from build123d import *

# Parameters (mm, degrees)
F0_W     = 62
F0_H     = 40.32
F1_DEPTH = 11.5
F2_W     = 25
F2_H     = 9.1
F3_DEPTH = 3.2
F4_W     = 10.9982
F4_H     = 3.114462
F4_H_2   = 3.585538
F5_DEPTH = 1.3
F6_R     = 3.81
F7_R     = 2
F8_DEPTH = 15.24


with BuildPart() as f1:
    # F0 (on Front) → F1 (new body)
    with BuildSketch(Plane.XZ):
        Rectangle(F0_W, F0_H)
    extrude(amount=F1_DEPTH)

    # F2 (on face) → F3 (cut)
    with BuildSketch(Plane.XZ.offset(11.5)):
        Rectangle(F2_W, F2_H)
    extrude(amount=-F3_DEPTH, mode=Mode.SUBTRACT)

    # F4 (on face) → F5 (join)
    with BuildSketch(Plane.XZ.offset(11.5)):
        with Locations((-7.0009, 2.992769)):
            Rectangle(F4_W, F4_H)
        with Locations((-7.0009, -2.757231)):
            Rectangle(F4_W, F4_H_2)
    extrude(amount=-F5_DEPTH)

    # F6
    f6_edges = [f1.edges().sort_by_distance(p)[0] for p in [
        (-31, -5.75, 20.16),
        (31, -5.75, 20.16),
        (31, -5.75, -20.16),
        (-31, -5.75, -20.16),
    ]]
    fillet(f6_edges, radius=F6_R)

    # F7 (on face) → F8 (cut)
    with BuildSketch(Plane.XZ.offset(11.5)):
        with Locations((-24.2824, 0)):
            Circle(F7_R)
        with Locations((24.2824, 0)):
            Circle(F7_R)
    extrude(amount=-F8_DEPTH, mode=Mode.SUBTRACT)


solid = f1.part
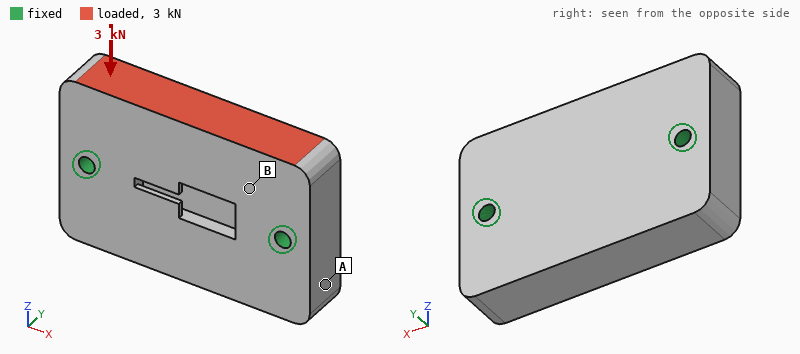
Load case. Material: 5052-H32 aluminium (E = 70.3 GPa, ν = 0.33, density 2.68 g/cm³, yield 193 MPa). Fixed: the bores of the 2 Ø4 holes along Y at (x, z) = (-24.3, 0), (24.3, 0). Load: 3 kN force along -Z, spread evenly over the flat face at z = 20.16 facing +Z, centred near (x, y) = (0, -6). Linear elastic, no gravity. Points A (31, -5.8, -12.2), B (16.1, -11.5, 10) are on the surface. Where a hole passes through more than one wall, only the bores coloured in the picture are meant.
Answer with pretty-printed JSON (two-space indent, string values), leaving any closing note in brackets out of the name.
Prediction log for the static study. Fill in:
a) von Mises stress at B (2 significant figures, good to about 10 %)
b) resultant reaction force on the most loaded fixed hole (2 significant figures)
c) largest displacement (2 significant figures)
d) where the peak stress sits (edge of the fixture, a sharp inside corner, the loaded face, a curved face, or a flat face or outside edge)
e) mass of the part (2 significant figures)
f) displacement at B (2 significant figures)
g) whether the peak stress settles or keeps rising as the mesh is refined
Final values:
{
  "von Mises stress at B": "6.8 MPa",
  "resultant reaction force on the most loaded fixed hole": "1.5 kN",
  "largest displacement": "3.8 µm",
  "where the peak stress sits": "edge of the fixture",
  "mass of the part": "74 g",
  "displacement at B": "2.0 µm",
  "whether the peak stress settles or keeps rising as the mesh is refined": "keeps rising"
}
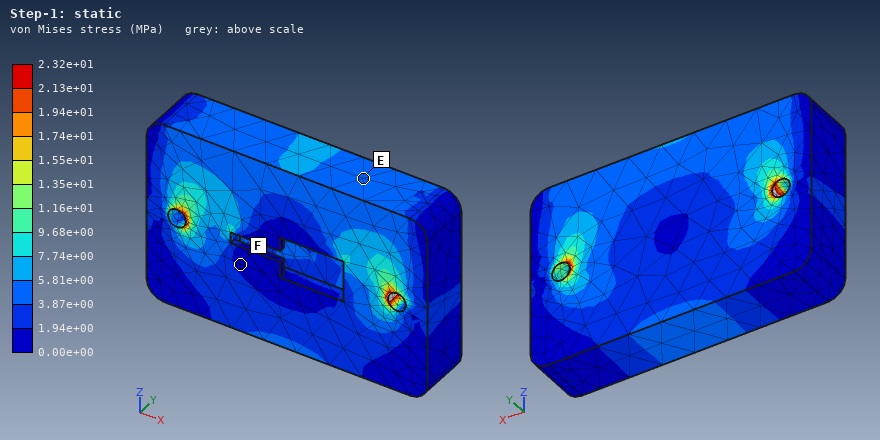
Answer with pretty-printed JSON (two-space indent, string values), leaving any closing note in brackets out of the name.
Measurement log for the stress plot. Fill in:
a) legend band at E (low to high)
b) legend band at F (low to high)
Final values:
{
  "legend band at E": "3.87e+00 to 5.81e+00 MPa",
  "legend band at F": "0.00e+00 to 1.94e+00 MPa"
}
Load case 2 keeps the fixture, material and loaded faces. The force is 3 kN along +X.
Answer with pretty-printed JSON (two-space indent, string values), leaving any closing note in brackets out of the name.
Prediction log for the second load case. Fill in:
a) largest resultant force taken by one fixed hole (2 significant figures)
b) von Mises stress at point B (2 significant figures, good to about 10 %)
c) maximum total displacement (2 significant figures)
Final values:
{
  "largest resultant force taken by one fixed hole": "1.9 kN",
  "von Mises stress at point B": "9.3 MPa",
  "maximum total displacement": "6.0 µm"
}
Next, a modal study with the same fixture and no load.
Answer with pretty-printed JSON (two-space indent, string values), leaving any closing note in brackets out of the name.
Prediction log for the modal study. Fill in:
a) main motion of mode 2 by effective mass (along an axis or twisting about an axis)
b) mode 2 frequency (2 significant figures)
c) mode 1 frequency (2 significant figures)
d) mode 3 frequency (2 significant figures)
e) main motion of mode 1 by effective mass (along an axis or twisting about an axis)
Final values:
{
  "main motion of mode 2 by effective mass": "along Y",
  "mode 2 frequency": "13 kHz",
  "mode 1 frequency": "11 kHz",
  "mode 3 frequency": "20 kHz",
  "main motion of mode 1 by effective mass": "twisting about X"
}
